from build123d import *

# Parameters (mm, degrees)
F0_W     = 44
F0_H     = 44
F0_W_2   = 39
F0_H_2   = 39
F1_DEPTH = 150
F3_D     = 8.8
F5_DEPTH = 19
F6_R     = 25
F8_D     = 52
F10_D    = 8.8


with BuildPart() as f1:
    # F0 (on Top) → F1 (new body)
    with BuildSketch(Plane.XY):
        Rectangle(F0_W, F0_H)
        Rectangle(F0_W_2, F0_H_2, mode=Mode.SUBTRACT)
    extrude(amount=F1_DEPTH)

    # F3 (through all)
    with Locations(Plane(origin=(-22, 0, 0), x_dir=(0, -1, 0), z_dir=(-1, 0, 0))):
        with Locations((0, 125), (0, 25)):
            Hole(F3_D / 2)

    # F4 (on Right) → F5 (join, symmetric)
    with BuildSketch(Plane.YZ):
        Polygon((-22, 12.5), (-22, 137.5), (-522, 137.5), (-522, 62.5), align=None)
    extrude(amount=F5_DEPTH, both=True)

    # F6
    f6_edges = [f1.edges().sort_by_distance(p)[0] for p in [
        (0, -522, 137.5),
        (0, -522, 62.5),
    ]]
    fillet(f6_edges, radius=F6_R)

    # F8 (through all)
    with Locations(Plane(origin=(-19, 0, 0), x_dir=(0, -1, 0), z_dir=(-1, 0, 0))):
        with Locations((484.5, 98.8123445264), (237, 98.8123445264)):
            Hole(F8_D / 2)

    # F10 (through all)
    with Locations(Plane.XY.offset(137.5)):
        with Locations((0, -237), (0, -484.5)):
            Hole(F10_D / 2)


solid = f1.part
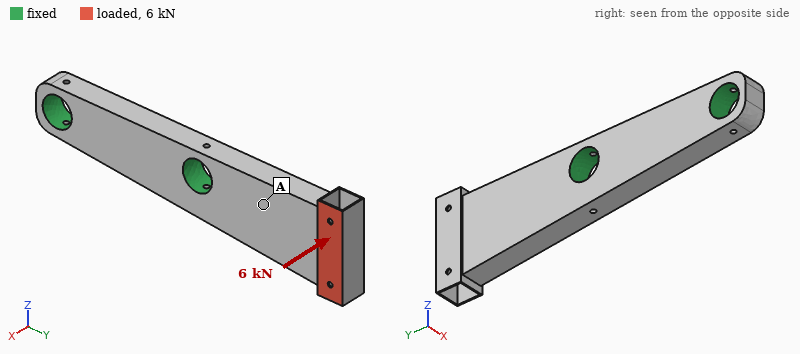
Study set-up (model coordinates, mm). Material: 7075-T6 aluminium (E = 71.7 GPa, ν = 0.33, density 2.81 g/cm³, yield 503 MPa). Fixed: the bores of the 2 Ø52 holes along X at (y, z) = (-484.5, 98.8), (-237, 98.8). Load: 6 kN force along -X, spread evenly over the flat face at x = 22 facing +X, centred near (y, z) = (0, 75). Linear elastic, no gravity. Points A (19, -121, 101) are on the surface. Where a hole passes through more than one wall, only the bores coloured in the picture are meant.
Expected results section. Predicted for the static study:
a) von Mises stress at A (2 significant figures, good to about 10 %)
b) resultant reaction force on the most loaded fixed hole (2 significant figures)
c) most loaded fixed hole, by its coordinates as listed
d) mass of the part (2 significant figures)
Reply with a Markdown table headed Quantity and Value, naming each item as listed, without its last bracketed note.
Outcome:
| Quantity | Value |
|---|---|
| von Mises stress at A | 26 MPa |
| resultant reaction force on the most loaded fixed hole | 6.1 kN |
| most loaded fixed hole, by its coordinates as listed | (-237, 98.8) |
| mass of the part | 5.0 kg |
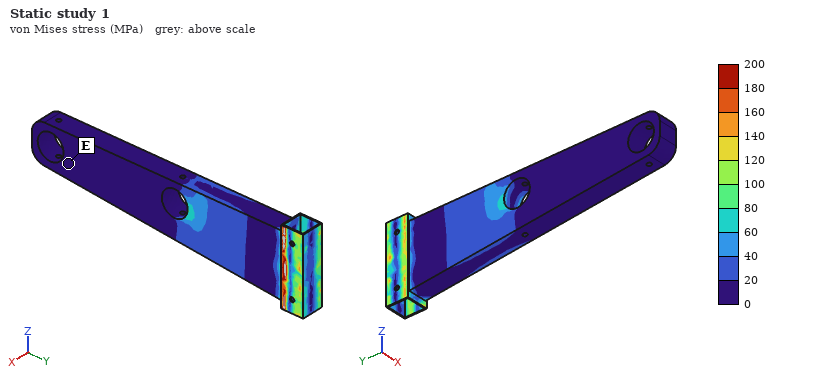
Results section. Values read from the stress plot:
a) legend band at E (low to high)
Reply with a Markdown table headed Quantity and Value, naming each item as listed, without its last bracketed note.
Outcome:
| Quantity | Value |
|---|---|
| legend band at E | 0 to 20 MPa |
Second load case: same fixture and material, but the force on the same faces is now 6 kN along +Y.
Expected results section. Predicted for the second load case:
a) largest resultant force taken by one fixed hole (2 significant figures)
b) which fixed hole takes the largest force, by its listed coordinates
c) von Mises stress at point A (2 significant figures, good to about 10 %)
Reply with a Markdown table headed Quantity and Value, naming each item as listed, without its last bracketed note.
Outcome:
| Quantity | Value |
|---|---|
| largest resultant force taken by one fixed hole | 5.7 kN |
| which fixed hole takes the largest force, by its listed coordinates | (-237, 98.8) |
| von Mises stress at point A | 6.0 MPa |
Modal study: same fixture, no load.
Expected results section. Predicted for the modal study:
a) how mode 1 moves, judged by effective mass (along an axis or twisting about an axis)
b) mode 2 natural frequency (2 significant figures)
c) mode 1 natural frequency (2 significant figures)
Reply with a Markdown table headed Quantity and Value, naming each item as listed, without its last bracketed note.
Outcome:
| Quantity | Value |
|---|---|
| how mode 1 moves, judged by effective mass | along X |
| mode 2 natural frequency | 1300 Hz |
| mode 1 natural frequency | 600 Hz |
